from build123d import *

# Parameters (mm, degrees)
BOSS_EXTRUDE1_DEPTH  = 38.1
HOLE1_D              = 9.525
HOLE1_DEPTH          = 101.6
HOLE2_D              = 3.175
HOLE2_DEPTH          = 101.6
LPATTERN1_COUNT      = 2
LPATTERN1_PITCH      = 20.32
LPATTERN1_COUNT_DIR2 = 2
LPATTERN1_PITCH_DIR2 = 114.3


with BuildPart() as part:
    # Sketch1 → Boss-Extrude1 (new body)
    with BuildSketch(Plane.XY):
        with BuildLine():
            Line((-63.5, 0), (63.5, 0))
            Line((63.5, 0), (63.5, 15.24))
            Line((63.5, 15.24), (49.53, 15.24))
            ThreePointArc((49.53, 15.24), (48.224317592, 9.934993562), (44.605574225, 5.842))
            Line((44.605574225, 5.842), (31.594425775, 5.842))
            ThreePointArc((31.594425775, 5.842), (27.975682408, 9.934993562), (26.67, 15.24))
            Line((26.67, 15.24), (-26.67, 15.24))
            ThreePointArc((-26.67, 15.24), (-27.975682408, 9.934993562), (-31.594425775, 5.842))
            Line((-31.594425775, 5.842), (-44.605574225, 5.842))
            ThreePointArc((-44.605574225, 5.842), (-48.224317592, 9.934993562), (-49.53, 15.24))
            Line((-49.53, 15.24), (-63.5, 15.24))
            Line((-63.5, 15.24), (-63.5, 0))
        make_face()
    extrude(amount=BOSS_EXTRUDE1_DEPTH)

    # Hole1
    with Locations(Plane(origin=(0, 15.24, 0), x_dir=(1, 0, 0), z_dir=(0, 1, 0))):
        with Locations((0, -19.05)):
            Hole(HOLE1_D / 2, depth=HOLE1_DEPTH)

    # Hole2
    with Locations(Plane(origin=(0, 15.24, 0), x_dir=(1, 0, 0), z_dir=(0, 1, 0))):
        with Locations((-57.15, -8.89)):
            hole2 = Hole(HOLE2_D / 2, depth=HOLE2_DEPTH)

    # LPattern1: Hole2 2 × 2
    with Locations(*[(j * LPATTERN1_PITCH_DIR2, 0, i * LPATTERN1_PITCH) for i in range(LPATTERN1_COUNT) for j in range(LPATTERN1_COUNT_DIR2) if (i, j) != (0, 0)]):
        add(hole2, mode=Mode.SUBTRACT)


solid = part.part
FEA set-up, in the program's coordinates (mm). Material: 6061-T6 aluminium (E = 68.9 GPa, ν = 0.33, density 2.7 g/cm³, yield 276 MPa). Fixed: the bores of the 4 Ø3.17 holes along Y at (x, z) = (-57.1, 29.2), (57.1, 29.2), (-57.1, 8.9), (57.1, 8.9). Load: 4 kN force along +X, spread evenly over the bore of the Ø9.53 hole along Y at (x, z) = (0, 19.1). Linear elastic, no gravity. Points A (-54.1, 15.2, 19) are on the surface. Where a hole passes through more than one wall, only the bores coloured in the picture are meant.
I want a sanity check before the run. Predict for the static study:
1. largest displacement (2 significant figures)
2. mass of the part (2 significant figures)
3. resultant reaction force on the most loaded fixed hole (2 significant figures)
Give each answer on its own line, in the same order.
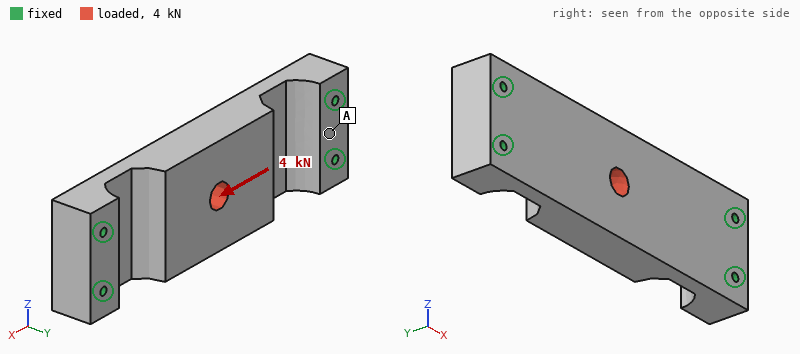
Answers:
8.5 µm
160 g
1.0 kN
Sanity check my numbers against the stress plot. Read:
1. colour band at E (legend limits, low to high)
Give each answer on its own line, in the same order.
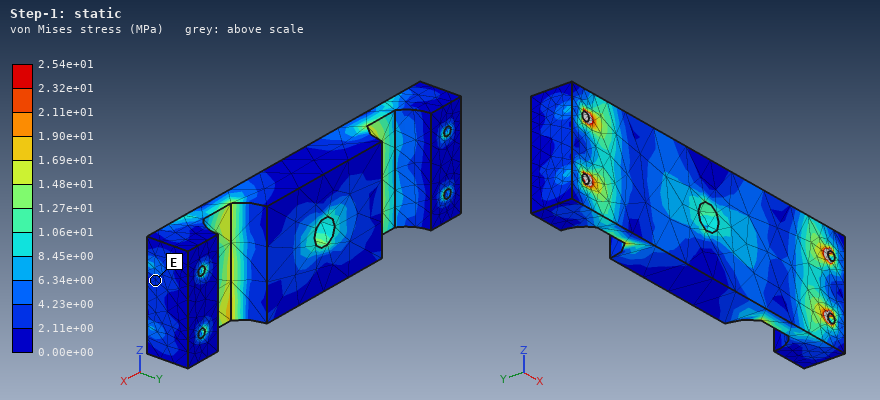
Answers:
2.11e+00 to 4.23e+00 MPa
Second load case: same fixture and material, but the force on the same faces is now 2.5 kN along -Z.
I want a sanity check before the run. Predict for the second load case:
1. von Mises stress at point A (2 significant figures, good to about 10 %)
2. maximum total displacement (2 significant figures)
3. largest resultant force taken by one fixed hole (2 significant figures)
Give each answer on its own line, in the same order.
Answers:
7.0 MPa
34 µm
1.4 kN
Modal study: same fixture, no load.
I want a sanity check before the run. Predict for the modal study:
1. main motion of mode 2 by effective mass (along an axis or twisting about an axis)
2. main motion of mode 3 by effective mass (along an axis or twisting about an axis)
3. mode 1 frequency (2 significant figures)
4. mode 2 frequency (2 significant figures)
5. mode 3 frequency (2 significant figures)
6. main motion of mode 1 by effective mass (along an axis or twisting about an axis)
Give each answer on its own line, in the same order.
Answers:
along Z
along Z
3800 Hz
4500 Hz
8200 Hz
along Y
